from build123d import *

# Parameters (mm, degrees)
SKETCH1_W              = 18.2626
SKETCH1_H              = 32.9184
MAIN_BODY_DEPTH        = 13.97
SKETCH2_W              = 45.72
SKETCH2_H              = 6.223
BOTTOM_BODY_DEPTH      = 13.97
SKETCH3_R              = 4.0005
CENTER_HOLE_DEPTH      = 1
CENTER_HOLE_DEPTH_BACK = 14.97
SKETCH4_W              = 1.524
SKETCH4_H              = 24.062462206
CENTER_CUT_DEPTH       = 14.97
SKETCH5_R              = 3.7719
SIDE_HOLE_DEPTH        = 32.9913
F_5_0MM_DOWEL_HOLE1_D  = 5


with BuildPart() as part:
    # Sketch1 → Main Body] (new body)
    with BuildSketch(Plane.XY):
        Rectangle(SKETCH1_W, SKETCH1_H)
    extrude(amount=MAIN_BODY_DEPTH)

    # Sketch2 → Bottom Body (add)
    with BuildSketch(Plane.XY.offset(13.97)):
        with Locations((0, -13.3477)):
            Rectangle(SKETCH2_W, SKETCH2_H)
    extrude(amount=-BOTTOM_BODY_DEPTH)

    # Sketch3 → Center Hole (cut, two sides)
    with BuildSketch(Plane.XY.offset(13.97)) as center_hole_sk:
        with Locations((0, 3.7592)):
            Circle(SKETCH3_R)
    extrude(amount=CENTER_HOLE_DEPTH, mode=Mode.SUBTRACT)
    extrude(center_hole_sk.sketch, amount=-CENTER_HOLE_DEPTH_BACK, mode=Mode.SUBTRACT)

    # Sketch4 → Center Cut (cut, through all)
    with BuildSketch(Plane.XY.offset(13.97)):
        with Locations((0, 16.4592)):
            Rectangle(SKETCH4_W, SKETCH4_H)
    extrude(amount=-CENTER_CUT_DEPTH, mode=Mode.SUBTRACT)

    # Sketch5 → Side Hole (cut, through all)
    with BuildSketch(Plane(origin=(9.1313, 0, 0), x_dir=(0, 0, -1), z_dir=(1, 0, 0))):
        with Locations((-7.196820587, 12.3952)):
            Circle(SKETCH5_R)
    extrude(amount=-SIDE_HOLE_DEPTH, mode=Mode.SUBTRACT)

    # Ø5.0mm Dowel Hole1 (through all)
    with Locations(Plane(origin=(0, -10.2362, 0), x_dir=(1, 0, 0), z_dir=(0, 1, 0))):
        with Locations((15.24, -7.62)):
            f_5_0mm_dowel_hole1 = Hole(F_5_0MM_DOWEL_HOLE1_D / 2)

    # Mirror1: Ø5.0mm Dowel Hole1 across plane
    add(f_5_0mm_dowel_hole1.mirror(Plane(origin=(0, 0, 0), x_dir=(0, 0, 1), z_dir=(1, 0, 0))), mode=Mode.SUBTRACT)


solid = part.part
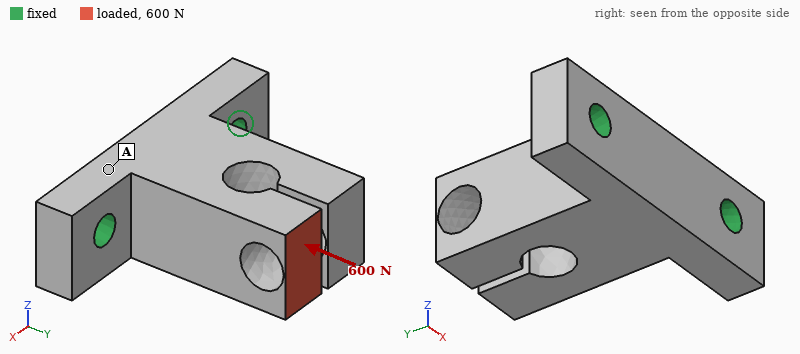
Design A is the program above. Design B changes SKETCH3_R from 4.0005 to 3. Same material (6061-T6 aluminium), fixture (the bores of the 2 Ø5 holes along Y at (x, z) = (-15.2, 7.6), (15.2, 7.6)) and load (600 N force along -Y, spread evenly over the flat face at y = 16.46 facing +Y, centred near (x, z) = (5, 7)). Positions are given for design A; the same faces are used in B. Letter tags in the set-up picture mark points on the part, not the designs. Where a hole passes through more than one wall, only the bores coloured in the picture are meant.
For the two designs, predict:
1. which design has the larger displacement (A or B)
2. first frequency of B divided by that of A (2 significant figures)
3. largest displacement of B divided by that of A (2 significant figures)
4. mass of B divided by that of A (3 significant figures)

A
0.98
0.79
1.03
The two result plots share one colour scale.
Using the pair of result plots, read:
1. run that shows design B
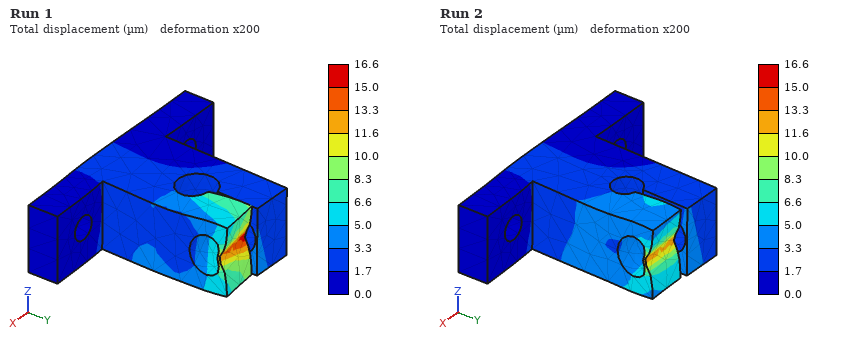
Run 2
